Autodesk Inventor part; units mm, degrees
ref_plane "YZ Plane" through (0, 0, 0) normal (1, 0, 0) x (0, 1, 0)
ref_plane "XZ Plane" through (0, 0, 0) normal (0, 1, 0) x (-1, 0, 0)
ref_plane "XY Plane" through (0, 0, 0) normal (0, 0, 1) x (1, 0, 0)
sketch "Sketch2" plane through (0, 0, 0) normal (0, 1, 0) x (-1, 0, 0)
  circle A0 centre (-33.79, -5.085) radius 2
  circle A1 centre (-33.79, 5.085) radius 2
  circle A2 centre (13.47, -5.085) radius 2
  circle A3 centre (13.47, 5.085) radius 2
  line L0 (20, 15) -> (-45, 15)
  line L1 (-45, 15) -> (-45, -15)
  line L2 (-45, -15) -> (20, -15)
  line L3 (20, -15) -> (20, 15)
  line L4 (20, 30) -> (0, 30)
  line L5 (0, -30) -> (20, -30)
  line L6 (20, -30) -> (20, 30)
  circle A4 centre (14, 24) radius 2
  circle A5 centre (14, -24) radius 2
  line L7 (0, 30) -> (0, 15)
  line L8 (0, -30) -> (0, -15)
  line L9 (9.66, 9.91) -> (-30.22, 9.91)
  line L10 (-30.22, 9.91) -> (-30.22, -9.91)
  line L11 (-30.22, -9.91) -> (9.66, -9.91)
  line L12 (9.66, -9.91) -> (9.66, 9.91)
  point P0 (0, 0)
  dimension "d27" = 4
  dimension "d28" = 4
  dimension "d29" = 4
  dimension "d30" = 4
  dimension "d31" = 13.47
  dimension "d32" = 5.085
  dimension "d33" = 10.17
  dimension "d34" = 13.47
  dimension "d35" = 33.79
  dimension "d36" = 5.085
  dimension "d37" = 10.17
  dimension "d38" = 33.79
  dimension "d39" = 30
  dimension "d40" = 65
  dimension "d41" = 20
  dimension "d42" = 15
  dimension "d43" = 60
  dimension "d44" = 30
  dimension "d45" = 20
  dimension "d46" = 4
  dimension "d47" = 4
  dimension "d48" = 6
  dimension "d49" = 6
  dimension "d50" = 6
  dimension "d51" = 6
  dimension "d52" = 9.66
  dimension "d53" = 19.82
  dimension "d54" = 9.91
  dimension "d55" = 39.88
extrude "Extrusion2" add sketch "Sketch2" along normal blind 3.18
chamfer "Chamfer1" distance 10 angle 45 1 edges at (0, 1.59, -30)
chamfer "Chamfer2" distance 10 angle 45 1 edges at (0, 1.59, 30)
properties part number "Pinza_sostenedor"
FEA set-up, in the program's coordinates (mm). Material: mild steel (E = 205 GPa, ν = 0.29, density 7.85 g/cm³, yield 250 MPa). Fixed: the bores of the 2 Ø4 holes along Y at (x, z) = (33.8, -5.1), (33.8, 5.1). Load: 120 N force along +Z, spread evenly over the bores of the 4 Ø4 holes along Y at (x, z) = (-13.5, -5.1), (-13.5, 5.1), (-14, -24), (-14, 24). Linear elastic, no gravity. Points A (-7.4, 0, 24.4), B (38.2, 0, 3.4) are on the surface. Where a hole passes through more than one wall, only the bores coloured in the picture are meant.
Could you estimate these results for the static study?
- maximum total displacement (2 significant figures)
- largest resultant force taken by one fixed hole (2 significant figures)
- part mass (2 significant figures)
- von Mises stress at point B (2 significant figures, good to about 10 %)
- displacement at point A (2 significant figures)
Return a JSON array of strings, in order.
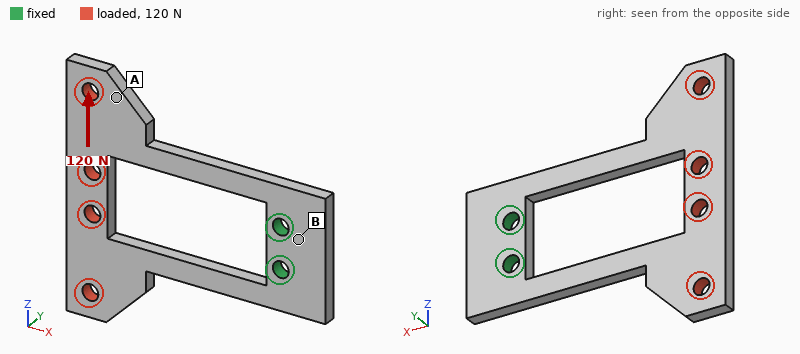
["62 µm", "340 N", "40 g", "15 MPa", "54 µm"]
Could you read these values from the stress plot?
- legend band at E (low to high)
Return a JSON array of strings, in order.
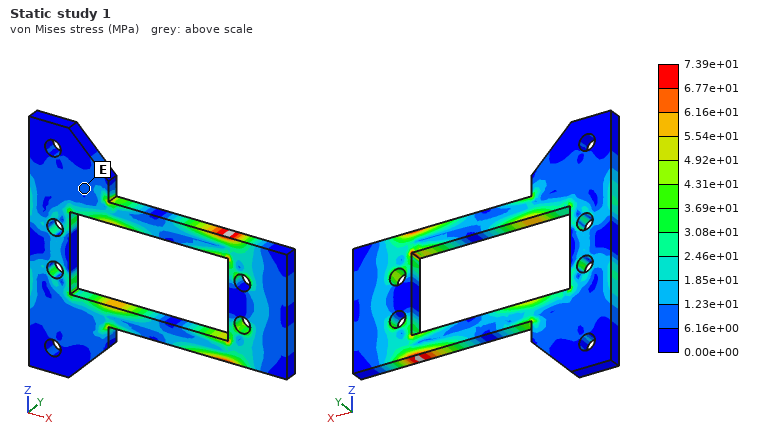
["6.16e+00 to 1.23e+01 MPa"]
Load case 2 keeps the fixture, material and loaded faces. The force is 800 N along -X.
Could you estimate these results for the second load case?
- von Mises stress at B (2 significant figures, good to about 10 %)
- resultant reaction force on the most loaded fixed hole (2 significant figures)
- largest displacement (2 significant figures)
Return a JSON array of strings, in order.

["5.2 MPa", "430 N", "9.9 µm"]
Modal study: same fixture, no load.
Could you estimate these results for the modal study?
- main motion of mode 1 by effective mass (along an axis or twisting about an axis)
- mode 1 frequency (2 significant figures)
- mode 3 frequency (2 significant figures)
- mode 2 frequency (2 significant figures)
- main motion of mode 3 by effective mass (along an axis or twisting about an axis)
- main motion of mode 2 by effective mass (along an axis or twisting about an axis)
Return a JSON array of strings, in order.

["along Y", "430 Hz", "1500 Hz", "900 Hz", "along Z", "twisting about X"]
